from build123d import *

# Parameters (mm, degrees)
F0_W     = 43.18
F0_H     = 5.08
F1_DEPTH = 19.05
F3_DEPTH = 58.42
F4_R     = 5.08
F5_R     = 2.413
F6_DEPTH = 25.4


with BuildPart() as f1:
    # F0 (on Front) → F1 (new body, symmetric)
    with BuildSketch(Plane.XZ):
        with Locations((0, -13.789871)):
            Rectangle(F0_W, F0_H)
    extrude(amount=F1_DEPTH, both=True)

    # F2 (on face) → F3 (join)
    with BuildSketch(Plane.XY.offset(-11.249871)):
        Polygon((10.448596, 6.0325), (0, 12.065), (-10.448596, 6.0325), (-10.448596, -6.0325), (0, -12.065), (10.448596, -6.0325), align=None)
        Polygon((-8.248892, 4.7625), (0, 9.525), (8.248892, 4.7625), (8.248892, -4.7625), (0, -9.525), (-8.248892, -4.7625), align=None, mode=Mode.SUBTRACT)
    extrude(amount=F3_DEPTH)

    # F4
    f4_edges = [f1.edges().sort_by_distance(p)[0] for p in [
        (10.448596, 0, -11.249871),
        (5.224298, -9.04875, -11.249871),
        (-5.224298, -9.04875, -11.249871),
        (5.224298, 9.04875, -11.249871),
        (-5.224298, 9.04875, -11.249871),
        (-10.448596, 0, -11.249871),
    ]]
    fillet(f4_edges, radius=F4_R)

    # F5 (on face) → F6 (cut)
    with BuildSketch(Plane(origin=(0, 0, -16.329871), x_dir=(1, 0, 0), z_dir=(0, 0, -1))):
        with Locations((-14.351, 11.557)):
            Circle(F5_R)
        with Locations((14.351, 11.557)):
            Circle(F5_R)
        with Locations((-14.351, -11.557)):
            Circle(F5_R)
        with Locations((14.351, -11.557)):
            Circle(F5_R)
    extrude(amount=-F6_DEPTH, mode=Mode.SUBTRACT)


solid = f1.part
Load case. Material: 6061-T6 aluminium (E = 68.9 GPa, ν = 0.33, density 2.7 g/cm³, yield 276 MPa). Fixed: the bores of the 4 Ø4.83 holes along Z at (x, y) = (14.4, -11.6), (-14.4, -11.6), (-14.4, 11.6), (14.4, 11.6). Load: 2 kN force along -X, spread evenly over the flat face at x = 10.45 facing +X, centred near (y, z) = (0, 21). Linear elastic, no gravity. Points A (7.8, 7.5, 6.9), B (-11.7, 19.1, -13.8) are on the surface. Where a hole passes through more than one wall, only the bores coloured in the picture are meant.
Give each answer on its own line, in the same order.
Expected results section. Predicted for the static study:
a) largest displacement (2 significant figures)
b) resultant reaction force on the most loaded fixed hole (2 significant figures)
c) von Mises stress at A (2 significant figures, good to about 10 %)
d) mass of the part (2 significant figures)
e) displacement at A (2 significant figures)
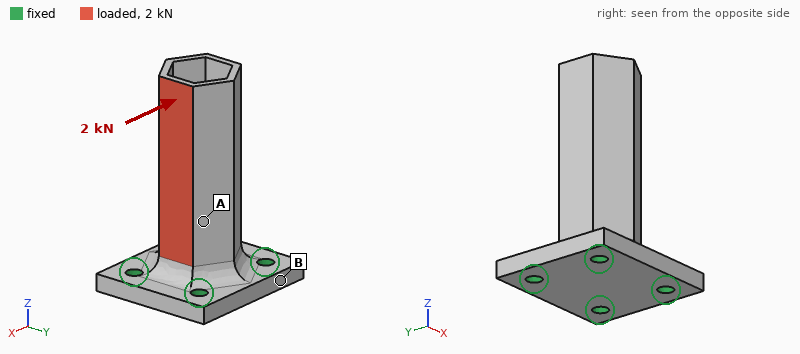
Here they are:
0.20 mm
1.5 kN
41 MPa
45 g
0.048 mm
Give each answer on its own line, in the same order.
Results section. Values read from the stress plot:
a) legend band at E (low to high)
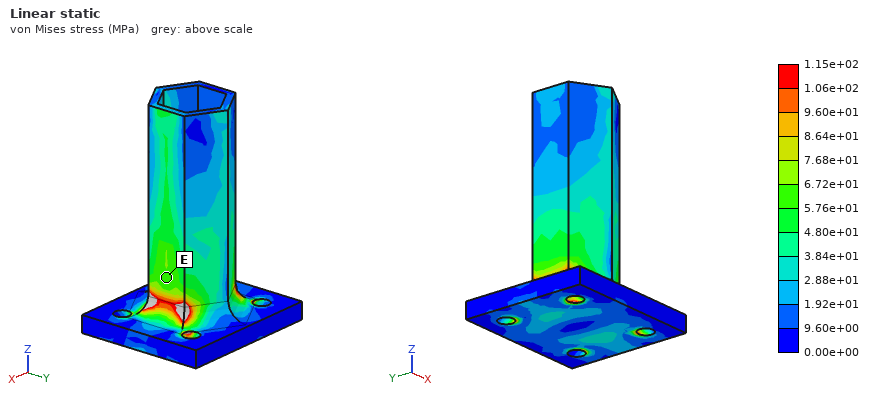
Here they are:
5.76e+01 to 6.72e+01 MPa
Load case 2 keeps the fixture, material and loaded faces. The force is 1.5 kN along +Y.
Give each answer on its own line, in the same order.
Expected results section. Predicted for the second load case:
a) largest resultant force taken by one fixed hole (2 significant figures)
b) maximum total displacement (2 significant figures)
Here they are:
1.3 kN
0.17 mm
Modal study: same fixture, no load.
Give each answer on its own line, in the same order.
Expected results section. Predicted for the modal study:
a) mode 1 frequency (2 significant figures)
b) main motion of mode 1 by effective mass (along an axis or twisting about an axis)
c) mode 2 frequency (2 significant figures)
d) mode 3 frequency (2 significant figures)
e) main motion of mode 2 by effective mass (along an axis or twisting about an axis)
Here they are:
4200 Hz
along Y
4500 Hz
13 kHz
along X
